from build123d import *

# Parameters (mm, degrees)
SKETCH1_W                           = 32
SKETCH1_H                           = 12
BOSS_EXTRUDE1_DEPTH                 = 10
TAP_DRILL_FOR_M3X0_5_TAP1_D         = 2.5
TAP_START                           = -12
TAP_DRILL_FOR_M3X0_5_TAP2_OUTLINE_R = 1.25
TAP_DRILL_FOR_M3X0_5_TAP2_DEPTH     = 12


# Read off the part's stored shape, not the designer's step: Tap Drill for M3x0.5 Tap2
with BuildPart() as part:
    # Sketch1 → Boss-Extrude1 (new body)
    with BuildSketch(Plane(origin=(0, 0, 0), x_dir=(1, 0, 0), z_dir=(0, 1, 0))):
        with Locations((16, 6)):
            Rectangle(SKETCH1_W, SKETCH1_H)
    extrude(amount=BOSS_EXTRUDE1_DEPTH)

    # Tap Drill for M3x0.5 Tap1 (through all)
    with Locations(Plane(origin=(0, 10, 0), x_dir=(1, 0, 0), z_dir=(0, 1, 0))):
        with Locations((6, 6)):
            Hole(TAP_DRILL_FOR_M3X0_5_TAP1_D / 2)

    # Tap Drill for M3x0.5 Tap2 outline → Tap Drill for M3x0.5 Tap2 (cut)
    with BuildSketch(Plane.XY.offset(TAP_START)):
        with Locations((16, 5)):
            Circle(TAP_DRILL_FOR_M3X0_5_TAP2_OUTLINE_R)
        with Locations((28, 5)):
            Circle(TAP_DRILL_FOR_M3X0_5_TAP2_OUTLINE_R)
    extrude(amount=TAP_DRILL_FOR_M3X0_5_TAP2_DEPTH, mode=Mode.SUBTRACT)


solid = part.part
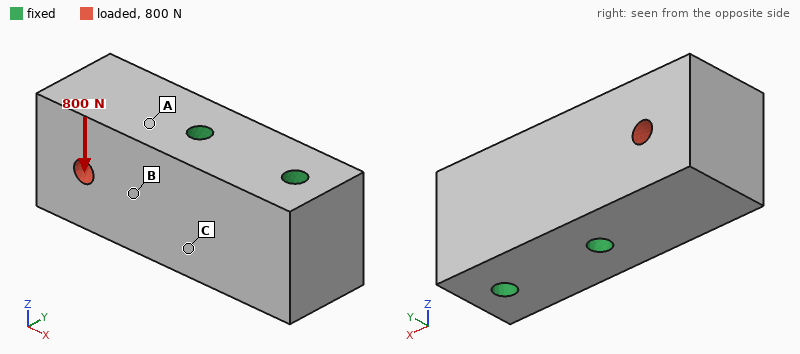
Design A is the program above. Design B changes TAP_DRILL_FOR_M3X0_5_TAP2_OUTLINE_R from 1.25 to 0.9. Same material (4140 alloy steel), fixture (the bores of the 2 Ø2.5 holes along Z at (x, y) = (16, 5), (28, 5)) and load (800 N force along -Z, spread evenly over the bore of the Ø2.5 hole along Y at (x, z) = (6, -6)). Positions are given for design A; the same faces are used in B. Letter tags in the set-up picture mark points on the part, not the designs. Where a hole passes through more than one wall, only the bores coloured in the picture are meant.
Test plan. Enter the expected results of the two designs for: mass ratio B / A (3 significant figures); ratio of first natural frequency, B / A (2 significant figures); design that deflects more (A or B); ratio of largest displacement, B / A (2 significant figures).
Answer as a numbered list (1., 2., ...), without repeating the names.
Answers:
1. 1.02
2. 0.94
3. B
4. 1.1
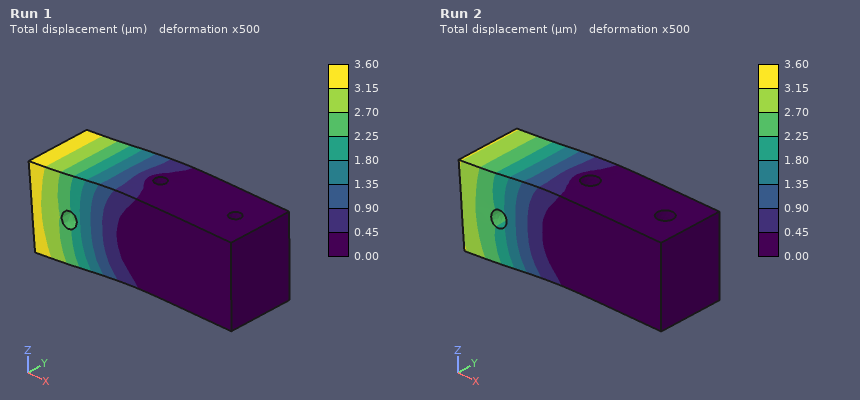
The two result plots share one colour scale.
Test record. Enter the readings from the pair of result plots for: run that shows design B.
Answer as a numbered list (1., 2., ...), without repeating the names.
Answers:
1. Run 1
